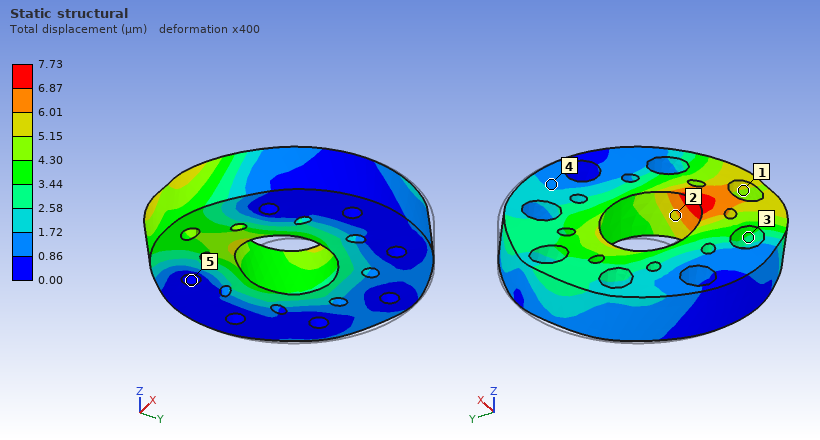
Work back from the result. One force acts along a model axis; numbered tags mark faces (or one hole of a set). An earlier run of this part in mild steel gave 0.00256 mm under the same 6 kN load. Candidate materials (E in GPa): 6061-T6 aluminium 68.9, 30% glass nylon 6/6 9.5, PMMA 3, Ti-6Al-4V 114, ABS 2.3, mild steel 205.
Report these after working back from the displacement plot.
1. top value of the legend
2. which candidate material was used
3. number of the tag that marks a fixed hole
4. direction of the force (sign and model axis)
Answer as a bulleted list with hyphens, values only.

- 7.73 µm
- 6061-T6 aluminium
- 5
- -Y
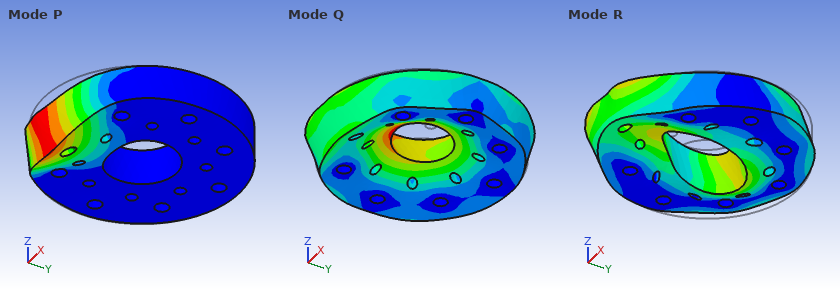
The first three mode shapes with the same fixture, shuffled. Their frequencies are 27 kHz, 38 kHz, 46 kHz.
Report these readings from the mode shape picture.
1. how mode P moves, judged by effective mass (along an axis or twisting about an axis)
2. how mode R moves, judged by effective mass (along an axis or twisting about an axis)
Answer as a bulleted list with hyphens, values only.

- along Z
- along Y
